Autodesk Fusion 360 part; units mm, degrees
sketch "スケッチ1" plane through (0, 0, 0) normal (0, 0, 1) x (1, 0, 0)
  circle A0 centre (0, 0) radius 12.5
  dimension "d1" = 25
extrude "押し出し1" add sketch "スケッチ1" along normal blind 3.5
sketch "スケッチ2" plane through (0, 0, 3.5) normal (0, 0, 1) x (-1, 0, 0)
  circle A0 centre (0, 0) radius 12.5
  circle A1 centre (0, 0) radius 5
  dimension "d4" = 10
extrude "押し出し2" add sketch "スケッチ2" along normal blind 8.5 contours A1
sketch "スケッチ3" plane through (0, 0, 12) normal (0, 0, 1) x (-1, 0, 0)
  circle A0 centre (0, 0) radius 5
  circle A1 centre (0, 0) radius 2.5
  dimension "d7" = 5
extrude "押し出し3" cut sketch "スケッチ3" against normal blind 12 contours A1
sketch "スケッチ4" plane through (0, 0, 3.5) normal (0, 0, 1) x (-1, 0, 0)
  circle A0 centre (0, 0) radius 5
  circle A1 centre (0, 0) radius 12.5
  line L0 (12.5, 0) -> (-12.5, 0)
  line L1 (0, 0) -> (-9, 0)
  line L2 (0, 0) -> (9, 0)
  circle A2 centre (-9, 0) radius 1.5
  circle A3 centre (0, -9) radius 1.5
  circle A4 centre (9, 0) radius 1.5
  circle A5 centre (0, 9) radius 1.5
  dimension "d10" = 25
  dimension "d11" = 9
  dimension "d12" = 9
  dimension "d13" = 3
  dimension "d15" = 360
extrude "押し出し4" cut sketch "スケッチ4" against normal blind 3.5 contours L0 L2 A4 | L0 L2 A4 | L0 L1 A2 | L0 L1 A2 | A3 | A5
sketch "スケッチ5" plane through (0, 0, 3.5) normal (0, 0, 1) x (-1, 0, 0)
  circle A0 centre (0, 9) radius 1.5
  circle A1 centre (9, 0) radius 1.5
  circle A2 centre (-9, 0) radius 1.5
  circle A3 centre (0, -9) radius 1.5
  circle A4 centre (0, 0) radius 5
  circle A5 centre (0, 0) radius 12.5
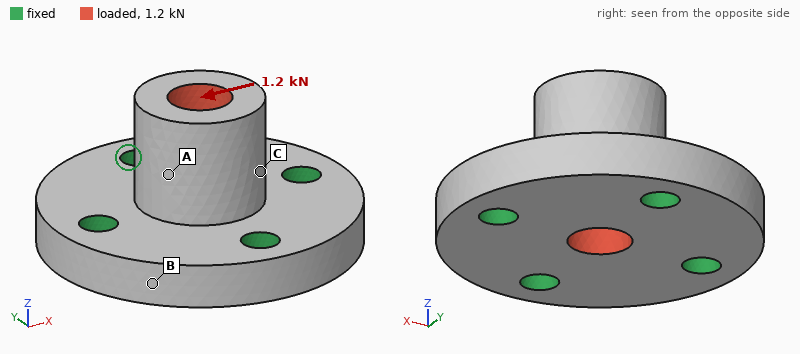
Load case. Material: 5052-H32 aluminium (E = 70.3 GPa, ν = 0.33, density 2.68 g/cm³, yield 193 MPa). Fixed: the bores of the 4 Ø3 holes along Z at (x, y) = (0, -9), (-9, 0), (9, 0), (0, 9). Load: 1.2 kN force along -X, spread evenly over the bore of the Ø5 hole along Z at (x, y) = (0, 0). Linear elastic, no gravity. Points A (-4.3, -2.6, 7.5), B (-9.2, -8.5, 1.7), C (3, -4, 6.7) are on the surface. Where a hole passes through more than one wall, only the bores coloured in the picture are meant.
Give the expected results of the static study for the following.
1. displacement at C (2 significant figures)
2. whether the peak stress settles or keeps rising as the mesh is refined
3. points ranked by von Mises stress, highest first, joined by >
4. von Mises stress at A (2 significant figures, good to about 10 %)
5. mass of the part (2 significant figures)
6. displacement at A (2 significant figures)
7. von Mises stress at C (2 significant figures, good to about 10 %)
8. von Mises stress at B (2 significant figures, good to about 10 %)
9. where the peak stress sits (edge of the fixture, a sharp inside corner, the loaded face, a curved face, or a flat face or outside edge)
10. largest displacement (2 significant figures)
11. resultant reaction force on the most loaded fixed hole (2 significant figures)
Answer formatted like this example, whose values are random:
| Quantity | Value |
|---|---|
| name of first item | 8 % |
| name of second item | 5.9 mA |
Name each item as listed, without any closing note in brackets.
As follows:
| Quantity | Value |
|---|---|
| displacement at C | 6.3 µm |
| whether the peak stress settles or keeps rising as the mesh is refined | keeps rising |
| points ranked by von Mises stress, highest first, joined by > | C > A > B |
| von Mises stress at A | 12 MPa |
| mass of the part | 5.5 g |
| displacement at A | 7.9 µm |
| von Mises stress at C | 18 MPa |
| von Mises stress at B | 5.2 MPa |
| where the peak stress sits | edge of the fixture |
| largest displacement | 13 µm |
| resultant reaction force on the most loaded fixed hole | 520 N |
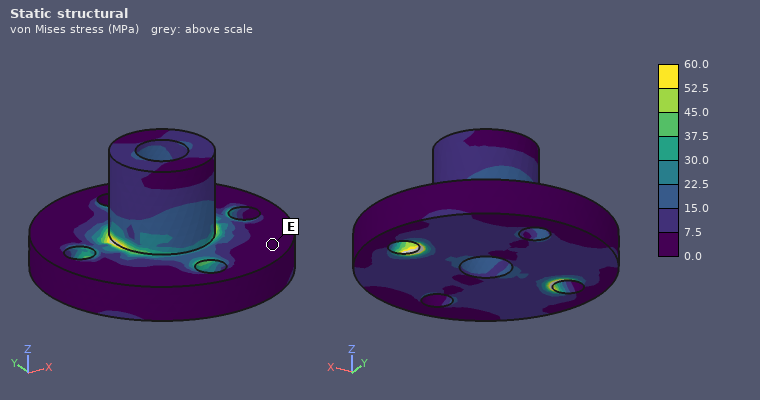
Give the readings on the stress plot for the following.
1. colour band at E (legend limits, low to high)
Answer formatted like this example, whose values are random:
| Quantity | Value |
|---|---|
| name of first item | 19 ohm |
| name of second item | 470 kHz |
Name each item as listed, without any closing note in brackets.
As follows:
| Quantity | Value |
|---|---|
| colour band at E | 0.0 to 7.5 MPa |
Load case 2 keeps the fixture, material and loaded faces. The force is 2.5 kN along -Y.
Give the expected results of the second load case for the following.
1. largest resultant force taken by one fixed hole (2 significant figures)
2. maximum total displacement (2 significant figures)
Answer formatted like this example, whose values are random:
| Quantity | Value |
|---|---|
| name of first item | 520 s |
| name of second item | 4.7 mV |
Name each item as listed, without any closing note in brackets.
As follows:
| Quantity | Value |
|---|---|
| largest resultant force taken by one fixed hole | 1.1 kN |
| maximum total displacement | 27 µm |
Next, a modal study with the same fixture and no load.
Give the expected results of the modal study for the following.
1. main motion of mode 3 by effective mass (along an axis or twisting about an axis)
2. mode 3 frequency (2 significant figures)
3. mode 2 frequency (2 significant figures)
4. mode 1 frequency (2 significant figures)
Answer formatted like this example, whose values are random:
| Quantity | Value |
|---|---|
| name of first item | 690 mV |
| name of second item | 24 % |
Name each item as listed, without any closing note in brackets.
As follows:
| Quantity | Value |
|---|---|
| main motion of mode 3 by effective mass | along Z |
| mode 3 frequency | 59 kHz |
| mode 2 frequency | 41 kHz |
| mode 1 frequency | 41 kHz |
